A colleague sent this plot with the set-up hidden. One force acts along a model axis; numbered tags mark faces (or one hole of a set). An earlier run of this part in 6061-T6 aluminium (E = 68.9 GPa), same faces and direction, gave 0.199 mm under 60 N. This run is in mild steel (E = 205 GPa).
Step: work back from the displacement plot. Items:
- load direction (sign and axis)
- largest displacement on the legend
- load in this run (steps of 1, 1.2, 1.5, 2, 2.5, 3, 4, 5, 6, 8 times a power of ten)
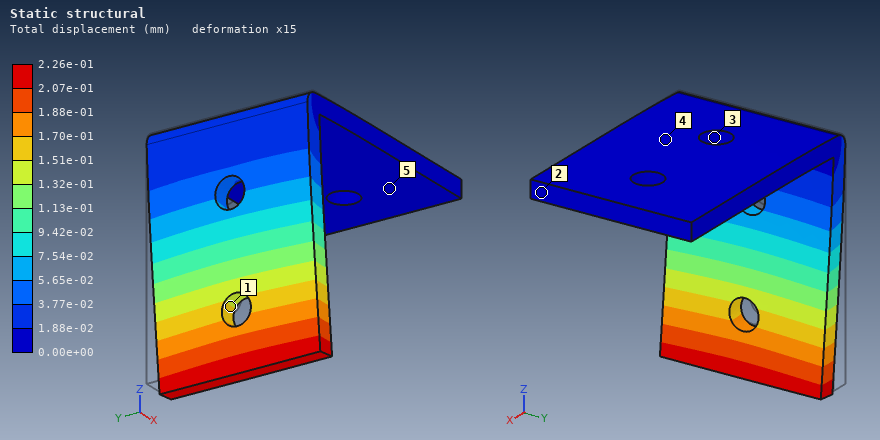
+X
2.26e-01 mm
200 N
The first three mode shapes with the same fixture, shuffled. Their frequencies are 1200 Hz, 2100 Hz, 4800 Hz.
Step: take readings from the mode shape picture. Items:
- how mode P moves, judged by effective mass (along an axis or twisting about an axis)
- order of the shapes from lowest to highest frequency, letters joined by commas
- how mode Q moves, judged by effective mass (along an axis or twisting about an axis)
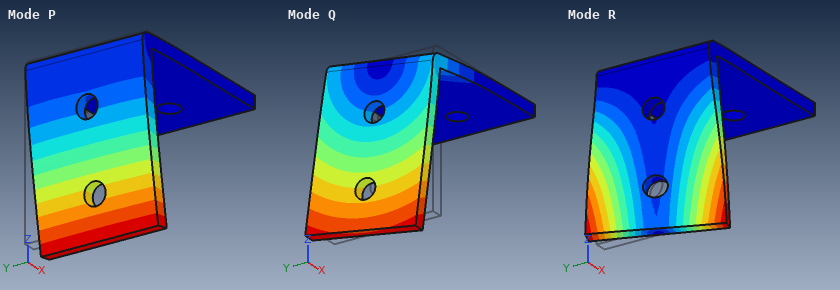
along X
P, Q, R
along Y
